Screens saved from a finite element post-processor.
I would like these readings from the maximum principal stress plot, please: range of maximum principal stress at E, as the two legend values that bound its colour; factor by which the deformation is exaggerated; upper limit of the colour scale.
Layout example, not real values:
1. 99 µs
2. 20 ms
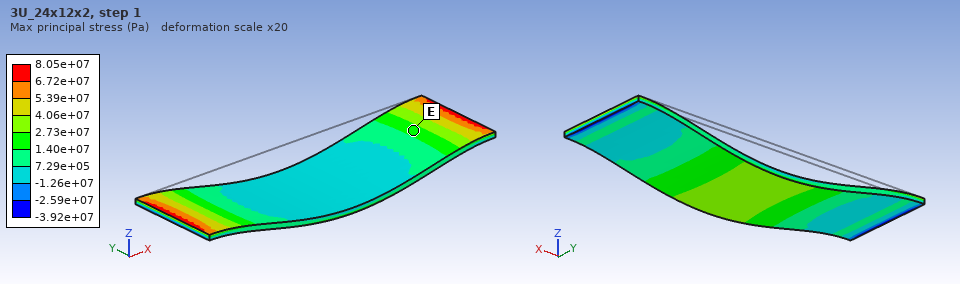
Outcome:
1. 1.40e+07 to 2.73e+07 Pa
2. 20
3. 8.05e+07 Pa
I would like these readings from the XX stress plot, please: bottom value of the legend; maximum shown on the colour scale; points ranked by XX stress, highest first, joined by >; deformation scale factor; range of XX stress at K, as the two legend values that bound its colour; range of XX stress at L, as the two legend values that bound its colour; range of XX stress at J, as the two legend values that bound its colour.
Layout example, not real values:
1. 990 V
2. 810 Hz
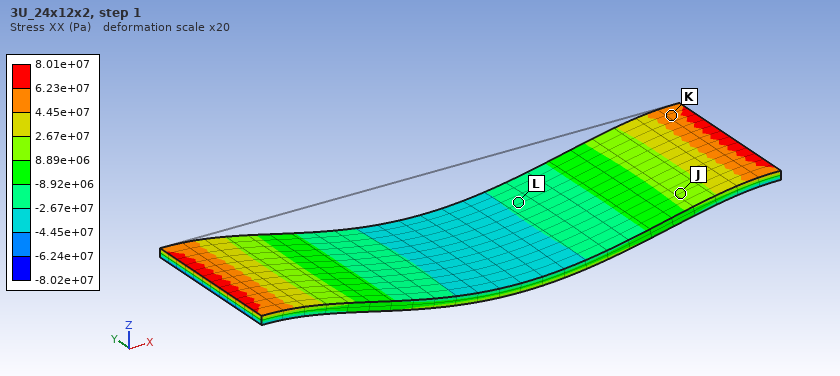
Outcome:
1. -8.02e+07 Pa
2. 8.01e+07 Pa
3. K > J > L
4. 20
5. 4.45e+07 to 6.23e+07 Pa
6. -2.67e+07 to -8.92e+06 Pa
7. 8.89e+06 to 2.67e+07 Pa
